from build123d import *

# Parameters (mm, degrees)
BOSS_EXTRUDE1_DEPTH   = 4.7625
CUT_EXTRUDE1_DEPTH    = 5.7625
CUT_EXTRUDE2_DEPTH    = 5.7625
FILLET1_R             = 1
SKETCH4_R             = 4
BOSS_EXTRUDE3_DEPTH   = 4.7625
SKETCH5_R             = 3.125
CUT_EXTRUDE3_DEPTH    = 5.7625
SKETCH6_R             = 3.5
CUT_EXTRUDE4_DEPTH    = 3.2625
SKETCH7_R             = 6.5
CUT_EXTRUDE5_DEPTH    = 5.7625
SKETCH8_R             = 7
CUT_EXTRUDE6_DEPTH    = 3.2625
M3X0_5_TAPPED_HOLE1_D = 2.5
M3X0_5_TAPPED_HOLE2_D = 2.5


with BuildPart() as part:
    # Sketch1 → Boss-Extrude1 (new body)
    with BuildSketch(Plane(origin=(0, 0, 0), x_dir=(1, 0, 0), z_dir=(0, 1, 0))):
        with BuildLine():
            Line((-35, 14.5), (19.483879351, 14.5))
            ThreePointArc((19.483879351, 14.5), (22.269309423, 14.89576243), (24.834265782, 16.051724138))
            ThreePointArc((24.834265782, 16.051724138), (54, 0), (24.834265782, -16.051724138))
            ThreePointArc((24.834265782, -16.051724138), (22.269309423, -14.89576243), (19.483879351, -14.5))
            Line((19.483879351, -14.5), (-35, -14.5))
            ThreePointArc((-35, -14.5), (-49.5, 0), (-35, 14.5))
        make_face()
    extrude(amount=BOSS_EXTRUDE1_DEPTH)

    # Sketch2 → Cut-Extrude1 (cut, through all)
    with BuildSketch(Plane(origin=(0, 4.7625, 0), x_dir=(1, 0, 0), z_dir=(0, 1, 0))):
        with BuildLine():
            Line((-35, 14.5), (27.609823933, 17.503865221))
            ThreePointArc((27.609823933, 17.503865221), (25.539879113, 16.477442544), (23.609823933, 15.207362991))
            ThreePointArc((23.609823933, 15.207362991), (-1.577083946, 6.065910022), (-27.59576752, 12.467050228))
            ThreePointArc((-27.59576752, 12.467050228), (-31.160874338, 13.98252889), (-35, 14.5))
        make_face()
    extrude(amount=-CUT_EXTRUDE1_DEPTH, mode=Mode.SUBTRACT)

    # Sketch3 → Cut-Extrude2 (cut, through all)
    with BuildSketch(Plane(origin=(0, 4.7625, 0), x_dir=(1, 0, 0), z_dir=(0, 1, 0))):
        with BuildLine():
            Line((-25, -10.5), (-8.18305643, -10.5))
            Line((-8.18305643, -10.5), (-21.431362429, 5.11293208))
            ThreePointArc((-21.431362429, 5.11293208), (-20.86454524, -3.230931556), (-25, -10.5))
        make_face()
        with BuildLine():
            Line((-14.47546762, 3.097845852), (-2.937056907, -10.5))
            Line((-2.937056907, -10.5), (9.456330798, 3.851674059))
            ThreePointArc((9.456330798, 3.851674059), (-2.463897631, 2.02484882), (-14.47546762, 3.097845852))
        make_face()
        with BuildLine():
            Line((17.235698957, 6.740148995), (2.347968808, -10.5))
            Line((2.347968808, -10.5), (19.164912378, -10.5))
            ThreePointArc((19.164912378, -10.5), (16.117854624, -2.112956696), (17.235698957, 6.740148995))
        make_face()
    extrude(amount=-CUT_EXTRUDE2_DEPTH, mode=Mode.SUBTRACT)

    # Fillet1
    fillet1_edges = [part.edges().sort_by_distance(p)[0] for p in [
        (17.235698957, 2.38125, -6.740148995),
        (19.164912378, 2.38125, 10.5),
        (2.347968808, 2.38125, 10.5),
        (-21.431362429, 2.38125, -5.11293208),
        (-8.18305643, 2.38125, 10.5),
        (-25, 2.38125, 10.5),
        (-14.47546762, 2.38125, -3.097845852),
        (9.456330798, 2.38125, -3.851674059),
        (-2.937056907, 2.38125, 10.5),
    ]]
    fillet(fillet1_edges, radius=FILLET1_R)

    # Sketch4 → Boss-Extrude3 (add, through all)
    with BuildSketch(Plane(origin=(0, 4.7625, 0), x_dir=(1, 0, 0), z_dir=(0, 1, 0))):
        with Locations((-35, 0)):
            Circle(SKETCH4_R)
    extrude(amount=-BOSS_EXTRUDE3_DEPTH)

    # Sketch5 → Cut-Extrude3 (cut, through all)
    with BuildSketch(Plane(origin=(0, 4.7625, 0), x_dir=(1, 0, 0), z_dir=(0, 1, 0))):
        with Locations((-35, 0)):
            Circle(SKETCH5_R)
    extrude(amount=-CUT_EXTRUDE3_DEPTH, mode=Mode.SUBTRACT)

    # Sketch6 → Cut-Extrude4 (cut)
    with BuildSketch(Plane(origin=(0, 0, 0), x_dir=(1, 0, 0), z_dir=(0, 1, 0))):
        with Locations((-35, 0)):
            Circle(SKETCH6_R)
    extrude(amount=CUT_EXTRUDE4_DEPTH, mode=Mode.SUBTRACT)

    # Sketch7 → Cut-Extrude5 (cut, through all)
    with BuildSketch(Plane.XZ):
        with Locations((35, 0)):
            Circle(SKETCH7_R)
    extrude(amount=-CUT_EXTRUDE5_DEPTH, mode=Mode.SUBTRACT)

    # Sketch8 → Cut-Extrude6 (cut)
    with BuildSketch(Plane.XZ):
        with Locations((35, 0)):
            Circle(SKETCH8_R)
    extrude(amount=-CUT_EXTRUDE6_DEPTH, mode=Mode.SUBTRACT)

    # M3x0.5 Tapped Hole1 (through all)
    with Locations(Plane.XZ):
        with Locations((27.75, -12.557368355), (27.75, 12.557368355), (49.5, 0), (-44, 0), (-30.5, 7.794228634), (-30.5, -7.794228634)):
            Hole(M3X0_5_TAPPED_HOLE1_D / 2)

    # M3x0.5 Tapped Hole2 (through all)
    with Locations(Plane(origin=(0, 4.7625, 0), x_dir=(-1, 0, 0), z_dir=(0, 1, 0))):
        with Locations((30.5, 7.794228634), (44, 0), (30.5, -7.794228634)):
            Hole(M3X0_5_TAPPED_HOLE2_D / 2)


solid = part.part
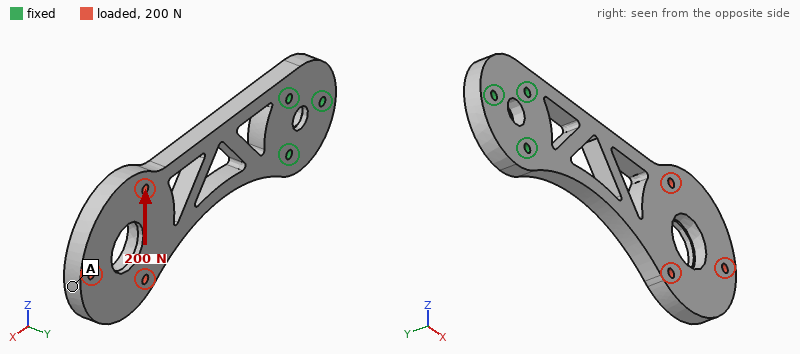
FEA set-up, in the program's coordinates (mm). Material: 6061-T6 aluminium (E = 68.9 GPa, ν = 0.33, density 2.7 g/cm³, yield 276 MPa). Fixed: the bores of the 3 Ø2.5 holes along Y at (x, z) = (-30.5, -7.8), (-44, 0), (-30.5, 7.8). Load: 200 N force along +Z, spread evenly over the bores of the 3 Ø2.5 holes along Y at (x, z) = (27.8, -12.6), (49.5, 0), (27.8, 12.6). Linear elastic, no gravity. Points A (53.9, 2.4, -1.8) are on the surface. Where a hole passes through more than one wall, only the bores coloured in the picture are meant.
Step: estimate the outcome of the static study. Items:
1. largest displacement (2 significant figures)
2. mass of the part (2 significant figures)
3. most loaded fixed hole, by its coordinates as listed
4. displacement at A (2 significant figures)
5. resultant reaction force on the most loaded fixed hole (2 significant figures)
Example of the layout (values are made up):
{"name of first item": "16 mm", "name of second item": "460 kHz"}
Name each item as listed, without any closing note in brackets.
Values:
{"largest displacement": "0.14 mm", "mass of the part": "27 g", "most loaded fixed hole, by its coordinates as listed": "(-30.5, -7.8)", "displacement at A": "0.14 mm", "resultant reaction force on the most loaded fixed hole": "720 N"}
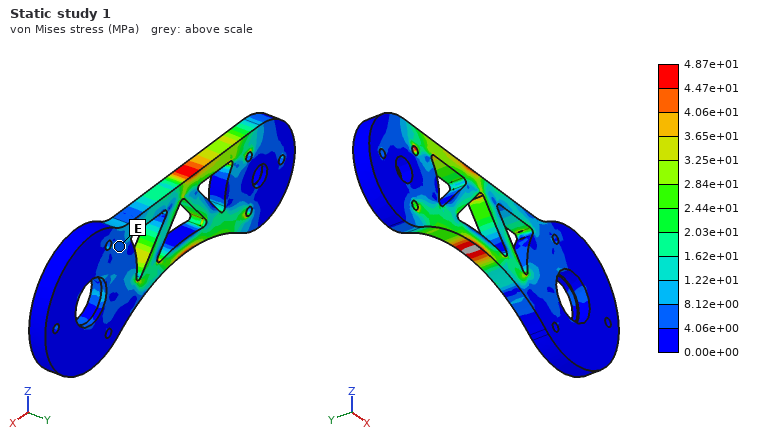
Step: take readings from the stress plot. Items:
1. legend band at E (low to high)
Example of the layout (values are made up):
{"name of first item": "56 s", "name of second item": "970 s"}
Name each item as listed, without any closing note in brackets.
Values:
{"legend band at E": "4.06e+00 to 8.12e+00 MPa"}
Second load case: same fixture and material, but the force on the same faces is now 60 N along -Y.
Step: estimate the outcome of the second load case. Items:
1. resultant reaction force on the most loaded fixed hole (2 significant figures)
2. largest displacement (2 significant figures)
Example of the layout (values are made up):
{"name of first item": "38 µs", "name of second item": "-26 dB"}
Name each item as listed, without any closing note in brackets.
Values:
{"resultant reaction force on the most loaded fixed hole": "58 N", "largest displacement": "1.1 mm"}
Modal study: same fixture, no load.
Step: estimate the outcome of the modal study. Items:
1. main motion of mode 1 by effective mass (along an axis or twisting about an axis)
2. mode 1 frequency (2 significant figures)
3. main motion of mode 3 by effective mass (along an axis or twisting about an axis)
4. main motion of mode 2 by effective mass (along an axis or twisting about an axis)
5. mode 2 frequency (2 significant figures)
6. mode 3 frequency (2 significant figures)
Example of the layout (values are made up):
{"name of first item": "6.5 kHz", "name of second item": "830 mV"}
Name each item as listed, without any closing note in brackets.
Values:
{"main motion of mode 1 by effective mass": "along Y", "mode 1 frequency": "380 Hz", "main motion of mode 3 by effective mass": "along Z", "main motion of mode 2 by effective mass": "twisting about X", "mode 2 frequency": "1600 Hz", "mode 3 frequency": "1800 Hz"}
